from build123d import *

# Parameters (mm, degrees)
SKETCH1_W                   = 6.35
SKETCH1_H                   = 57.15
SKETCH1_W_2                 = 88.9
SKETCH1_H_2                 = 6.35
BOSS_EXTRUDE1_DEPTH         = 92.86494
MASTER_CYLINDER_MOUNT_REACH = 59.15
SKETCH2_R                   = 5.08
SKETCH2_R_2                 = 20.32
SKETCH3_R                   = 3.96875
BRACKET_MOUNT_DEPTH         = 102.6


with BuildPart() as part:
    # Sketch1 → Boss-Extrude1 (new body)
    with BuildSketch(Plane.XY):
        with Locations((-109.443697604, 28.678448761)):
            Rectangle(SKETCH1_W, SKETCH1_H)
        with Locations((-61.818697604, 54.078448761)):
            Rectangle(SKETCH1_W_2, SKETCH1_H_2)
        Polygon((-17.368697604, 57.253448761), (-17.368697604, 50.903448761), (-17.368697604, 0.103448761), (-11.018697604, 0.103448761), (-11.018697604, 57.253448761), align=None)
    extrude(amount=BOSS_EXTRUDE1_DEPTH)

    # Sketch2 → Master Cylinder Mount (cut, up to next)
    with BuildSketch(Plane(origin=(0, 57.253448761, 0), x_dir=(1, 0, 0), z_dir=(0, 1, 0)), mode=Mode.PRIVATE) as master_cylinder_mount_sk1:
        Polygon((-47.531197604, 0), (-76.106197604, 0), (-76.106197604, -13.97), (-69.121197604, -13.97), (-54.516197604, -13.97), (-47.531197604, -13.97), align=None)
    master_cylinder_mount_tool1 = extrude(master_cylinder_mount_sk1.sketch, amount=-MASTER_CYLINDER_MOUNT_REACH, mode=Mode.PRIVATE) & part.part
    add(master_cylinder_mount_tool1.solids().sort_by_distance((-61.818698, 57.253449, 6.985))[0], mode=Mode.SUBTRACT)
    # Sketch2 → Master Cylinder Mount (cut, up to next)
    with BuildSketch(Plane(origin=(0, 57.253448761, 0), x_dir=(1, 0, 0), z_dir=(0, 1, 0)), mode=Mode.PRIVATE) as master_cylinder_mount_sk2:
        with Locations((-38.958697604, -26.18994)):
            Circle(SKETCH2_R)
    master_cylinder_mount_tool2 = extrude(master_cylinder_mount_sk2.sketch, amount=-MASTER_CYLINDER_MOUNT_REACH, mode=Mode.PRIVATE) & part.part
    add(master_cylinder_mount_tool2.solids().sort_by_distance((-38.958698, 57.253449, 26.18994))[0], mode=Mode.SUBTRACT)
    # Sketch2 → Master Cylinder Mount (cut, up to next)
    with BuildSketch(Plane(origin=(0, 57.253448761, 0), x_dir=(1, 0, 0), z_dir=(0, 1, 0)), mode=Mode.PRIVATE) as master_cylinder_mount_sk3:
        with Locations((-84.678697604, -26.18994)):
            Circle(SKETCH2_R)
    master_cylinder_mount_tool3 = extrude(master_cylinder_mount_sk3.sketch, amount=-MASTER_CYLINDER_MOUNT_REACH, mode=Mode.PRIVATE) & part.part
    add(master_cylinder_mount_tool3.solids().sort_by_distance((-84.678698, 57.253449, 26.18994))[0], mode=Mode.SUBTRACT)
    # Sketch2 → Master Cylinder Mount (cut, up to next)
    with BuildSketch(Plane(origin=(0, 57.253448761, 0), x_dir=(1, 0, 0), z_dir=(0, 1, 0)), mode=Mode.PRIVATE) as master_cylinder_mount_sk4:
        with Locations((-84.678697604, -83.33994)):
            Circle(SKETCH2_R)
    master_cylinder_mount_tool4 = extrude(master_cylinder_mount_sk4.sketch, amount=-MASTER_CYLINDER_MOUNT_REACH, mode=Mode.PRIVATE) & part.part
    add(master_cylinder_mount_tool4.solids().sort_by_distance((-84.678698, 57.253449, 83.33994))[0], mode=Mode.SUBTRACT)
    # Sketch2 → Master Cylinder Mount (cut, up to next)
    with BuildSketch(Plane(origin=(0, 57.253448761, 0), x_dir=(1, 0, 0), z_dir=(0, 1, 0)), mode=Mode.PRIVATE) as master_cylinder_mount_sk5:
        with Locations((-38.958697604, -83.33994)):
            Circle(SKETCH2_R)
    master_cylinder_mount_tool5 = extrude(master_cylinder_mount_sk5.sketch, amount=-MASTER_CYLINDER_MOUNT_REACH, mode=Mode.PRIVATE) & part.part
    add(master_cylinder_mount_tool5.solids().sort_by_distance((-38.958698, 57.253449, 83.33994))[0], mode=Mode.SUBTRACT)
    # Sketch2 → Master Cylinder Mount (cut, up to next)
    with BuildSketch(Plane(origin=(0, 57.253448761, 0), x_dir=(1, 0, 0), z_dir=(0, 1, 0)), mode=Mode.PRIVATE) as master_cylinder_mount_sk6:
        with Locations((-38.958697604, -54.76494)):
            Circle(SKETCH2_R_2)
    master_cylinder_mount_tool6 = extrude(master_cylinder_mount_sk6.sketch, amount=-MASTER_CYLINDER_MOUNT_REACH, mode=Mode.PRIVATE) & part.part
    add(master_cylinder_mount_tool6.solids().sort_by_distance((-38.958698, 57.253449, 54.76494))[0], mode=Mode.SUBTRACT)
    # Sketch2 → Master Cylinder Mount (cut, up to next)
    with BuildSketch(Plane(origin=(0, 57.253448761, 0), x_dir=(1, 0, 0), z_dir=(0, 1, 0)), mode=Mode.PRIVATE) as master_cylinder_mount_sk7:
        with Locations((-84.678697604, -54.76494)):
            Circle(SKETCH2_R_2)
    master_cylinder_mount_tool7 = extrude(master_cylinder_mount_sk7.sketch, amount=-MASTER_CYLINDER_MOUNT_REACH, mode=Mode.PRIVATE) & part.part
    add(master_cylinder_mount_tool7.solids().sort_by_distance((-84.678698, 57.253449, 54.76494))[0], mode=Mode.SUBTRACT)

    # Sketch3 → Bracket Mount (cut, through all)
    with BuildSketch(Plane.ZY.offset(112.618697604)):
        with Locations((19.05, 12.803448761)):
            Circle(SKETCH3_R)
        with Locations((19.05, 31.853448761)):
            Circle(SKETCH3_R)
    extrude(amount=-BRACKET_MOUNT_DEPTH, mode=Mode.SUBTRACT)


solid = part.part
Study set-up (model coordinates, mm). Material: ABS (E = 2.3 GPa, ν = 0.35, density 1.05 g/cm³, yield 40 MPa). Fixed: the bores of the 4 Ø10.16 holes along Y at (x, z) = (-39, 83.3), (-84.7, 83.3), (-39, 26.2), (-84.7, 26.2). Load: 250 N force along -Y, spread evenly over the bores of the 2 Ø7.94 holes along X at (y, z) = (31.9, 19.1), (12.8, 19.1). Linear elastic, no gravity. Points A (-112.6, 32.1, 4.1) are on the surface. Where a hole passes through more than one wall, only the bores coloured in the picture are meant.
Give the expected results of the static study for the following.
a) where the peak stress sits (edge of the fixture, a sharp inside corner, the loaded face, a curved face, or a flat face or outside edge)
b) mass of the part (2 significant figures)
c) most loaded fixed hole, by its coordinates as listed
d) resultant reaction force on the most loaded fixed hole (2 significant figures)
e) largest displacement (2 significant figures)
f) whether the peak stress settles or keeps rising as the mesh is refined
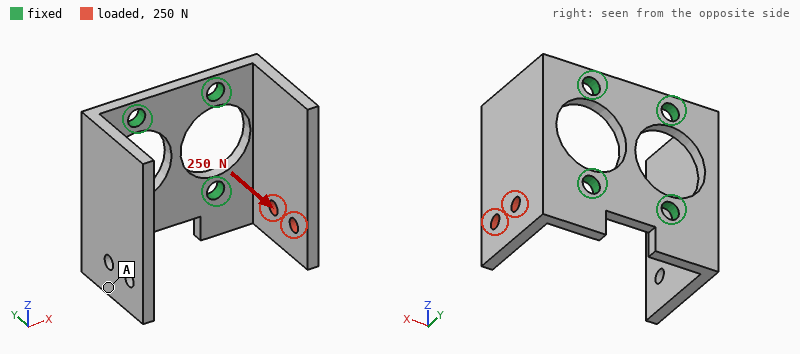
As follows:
edge of the fixture
100 g
(-39, 26.2)
260 N
1.7 mm
keeps rising
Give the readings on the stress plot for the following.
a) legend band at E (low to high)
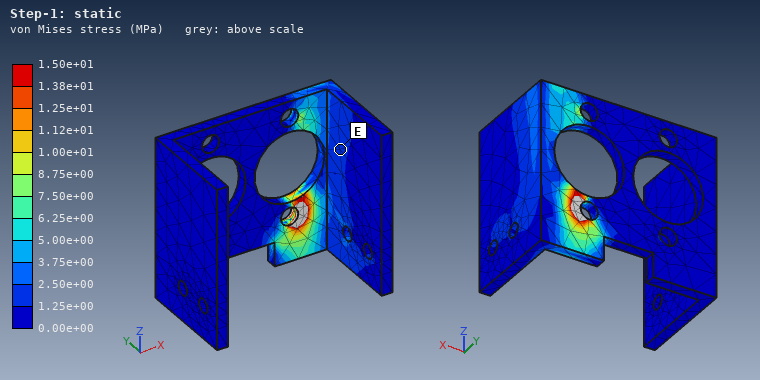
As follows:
1.25e+00 to 2.50e+00 MPa
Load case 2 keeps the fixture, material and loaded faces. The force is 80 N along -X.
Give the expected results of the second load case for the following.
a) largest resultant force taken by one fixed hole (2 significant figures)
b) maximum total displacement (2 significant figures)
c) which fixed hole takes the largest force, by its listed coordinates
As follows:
76 N
1.7 mm
(-39, 26.2)
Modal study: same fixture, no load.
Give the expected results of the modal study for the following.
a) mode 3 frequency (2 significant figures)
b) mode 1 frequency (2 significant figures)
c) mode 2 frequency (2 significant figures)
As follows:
590 Hz
270 Hz
270 Hz
